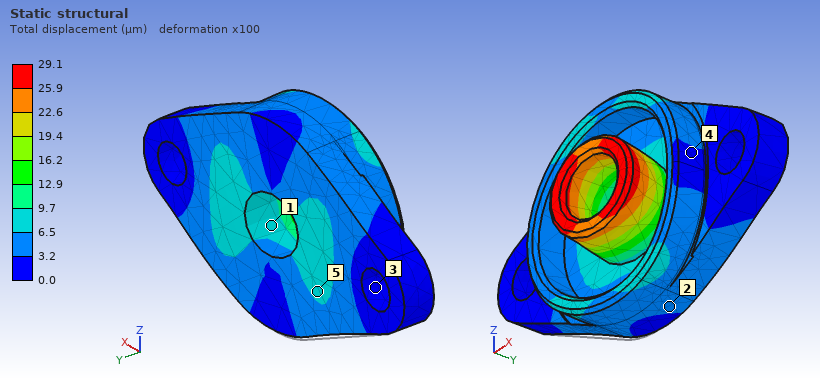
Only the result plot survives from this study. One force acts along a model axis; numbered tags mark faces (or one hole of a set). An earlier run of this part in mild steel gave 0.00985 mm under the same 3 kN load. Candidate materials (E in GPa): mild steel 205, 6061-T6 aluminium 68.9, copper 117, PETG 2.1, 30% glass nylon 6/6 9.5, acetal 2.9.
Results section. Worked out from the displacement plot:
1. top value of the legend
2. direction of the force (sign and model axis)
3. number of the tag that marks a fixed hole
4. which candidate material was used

29.1 µm
+X
3
6061-T6 aluminium
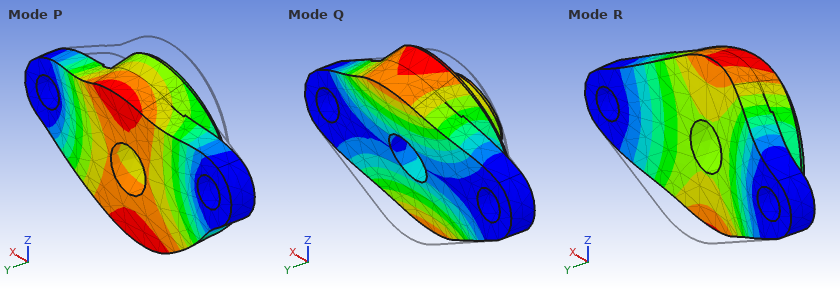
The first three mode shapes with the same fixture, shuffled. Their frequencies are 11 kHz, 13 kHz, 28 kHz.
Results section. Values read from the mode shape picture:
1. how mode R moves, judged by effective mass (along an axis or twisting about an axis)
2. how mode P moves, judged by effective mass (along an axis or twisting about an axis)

along Y
along Z
